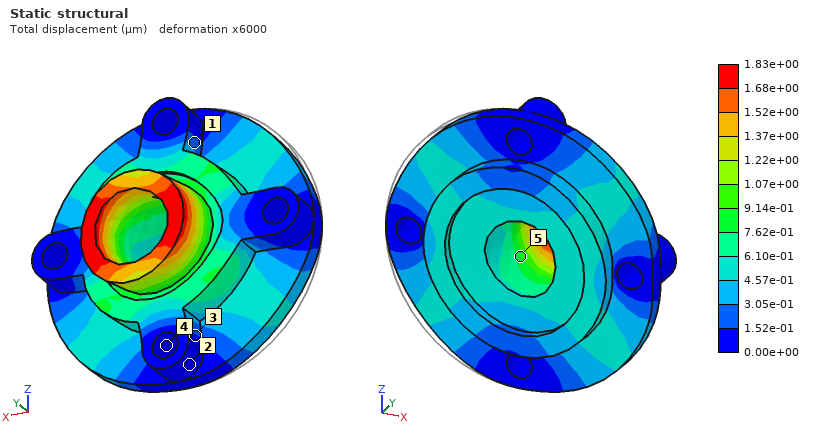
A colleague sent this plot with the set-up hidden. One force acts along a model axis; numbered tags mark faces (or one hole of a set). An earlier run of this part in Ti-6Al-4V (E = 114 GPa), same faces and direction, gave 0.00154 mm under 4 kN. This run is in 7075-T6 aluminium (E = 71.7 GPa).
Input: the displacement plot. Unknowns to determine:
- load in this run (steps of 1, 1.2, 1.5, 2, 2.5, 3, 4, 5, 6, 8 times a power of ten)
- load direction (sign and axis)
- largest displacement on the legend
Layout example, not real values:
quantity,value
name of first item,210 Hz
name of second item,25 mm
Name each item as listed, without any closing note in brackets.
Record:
quantity,value
load in this run,3 kN
load direction,+X
largest displacement on the legend,1.83e+00 µm
